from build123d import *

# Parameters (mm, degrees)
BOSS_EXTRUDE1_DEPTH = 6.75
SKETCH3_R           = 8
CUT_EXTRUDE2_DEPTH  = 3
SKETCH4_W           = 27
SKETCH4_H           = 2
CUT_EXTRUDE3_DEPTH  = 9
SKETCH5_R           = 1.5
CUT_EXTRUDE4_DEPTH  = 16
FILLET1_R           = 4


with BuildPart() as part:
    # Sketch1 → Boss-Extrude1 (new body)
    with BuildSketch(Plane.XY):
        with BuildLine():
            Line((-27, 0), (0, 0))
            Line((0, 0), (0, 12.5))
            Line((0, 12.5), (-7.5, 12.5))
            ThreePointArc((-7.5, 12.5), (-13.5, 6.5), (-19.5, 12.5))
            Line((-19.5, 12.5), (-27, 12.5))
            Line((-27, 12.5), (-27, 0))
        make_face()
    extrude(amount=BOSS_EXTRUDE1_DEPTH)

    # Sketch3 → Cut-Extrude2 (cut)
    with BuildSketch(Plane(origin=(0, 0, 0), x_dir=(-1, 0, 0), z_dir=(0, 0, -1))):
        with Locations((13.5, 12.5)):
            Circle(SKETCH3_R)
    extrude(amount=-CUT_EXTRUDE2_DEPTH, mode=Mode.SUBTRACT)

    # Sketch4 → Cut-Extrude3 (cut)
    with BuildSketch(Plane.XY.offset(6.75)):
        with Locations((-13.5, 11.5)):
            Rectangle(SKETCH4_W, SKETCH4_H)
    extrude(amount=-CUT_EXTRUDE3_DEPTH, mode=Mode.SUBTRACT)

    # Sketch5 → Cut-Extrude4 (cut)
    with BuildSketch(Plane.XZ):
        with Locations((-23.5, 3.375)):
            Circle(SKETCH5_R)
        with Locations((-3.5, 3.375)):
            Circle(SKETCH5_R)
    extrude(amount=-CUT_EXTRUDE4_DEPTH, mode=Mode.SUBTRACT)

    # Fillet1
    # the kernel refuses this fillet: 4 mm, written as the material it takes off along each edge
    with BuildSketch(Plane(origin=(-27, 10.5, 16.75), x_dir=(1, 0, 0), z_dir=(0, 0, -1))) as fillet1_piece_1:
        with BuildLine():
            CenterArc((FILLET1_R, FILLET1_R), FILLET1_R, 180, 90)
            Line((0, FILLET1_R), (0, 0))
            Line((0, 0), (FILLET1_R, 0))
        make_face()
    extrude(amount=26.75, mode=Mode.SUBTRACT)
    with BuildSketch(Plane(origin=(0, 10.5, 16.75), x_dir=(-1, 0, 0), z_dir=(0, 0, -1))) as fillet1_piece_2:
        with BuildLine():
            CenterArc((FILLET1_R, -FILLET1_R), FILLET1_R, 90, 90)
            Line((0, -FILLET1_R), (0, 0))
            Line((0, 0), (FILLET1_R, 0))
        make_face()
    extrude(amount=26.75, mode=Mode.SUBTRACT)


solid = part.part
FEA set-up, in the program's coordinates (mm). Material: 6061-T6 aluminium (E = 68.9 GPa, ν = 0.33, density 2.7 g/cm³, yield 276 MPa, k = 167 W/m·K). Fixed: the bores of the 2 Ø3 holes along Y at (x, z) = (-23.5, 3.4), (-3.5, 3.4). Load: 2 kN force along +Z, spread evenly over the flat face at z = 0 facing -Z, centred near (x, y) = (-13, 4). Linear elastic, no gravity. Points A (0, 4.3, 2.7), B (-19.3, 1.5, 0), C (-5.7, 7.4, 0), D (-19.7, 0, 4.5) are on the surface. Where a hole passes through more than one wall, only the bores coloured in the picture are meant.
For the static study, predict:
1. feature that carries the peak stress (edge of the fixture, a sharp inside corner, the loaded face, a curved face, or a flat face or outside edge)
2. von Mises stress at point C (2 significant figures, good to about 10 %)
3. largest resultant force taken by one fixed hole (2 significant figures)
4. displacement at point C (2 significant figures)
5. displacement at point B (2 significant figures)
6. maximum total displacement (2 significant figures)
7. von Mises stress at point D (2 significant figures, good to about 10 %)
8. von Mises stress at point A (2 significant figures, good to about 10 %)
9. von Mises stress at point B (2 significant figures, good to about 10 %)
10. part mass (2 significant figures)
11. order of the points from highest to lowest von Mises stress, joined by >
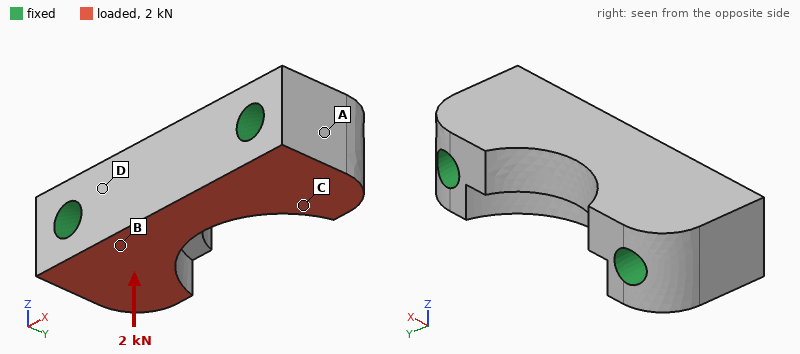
edge of the fixture
18 MPa
1.0 kN
1.2 µm
2.9 µm
5.3 µm
23 MPa
5.4 MPa
11 MPa
3.8 g
D > C > B > A
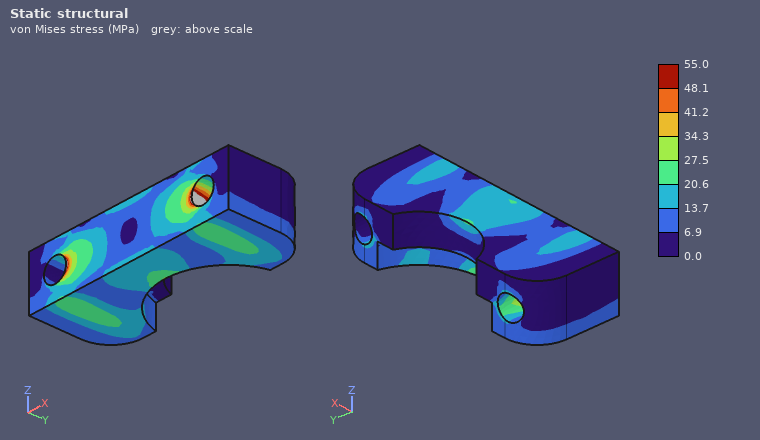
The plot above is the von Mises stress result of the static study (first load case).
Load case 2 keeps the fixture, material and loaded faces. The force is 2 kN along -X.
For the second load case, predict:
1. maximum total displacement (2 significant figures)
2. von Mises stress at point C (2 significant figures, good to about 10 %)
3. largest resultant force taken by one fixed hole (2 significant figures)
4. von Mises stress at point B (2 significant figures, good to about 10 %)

2.3 µm
19 MPa
1.0 kN
17 MPa
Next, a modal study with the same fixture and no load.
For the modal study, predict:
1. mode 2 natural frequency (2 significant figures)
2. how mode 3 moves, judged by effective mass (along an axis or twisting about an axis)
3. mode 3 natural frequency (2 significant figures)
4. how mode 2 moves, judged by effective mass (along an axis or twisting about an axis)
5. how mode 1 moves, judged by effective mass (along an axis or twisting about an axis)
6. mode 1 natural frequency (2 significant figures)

78 kHz
twisting about X
96 kHz
along Y
along Z
59 kHz
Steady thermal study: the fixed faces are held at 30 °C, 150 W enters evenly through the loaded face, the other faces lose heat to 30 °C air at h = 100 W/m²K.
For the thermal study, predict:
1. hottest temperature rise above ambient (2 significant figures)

31 K
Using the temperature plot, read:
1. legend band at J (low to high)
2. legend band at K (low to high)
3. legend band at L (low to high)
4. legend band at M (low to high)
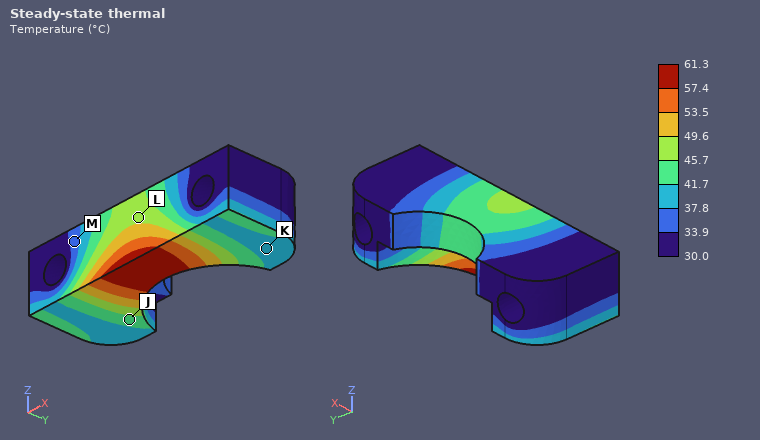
41.7 to 45.7 °C
37.8 to 41.7 °C
45.7 to 49.6 °C
33.9 to 37.8 °C
